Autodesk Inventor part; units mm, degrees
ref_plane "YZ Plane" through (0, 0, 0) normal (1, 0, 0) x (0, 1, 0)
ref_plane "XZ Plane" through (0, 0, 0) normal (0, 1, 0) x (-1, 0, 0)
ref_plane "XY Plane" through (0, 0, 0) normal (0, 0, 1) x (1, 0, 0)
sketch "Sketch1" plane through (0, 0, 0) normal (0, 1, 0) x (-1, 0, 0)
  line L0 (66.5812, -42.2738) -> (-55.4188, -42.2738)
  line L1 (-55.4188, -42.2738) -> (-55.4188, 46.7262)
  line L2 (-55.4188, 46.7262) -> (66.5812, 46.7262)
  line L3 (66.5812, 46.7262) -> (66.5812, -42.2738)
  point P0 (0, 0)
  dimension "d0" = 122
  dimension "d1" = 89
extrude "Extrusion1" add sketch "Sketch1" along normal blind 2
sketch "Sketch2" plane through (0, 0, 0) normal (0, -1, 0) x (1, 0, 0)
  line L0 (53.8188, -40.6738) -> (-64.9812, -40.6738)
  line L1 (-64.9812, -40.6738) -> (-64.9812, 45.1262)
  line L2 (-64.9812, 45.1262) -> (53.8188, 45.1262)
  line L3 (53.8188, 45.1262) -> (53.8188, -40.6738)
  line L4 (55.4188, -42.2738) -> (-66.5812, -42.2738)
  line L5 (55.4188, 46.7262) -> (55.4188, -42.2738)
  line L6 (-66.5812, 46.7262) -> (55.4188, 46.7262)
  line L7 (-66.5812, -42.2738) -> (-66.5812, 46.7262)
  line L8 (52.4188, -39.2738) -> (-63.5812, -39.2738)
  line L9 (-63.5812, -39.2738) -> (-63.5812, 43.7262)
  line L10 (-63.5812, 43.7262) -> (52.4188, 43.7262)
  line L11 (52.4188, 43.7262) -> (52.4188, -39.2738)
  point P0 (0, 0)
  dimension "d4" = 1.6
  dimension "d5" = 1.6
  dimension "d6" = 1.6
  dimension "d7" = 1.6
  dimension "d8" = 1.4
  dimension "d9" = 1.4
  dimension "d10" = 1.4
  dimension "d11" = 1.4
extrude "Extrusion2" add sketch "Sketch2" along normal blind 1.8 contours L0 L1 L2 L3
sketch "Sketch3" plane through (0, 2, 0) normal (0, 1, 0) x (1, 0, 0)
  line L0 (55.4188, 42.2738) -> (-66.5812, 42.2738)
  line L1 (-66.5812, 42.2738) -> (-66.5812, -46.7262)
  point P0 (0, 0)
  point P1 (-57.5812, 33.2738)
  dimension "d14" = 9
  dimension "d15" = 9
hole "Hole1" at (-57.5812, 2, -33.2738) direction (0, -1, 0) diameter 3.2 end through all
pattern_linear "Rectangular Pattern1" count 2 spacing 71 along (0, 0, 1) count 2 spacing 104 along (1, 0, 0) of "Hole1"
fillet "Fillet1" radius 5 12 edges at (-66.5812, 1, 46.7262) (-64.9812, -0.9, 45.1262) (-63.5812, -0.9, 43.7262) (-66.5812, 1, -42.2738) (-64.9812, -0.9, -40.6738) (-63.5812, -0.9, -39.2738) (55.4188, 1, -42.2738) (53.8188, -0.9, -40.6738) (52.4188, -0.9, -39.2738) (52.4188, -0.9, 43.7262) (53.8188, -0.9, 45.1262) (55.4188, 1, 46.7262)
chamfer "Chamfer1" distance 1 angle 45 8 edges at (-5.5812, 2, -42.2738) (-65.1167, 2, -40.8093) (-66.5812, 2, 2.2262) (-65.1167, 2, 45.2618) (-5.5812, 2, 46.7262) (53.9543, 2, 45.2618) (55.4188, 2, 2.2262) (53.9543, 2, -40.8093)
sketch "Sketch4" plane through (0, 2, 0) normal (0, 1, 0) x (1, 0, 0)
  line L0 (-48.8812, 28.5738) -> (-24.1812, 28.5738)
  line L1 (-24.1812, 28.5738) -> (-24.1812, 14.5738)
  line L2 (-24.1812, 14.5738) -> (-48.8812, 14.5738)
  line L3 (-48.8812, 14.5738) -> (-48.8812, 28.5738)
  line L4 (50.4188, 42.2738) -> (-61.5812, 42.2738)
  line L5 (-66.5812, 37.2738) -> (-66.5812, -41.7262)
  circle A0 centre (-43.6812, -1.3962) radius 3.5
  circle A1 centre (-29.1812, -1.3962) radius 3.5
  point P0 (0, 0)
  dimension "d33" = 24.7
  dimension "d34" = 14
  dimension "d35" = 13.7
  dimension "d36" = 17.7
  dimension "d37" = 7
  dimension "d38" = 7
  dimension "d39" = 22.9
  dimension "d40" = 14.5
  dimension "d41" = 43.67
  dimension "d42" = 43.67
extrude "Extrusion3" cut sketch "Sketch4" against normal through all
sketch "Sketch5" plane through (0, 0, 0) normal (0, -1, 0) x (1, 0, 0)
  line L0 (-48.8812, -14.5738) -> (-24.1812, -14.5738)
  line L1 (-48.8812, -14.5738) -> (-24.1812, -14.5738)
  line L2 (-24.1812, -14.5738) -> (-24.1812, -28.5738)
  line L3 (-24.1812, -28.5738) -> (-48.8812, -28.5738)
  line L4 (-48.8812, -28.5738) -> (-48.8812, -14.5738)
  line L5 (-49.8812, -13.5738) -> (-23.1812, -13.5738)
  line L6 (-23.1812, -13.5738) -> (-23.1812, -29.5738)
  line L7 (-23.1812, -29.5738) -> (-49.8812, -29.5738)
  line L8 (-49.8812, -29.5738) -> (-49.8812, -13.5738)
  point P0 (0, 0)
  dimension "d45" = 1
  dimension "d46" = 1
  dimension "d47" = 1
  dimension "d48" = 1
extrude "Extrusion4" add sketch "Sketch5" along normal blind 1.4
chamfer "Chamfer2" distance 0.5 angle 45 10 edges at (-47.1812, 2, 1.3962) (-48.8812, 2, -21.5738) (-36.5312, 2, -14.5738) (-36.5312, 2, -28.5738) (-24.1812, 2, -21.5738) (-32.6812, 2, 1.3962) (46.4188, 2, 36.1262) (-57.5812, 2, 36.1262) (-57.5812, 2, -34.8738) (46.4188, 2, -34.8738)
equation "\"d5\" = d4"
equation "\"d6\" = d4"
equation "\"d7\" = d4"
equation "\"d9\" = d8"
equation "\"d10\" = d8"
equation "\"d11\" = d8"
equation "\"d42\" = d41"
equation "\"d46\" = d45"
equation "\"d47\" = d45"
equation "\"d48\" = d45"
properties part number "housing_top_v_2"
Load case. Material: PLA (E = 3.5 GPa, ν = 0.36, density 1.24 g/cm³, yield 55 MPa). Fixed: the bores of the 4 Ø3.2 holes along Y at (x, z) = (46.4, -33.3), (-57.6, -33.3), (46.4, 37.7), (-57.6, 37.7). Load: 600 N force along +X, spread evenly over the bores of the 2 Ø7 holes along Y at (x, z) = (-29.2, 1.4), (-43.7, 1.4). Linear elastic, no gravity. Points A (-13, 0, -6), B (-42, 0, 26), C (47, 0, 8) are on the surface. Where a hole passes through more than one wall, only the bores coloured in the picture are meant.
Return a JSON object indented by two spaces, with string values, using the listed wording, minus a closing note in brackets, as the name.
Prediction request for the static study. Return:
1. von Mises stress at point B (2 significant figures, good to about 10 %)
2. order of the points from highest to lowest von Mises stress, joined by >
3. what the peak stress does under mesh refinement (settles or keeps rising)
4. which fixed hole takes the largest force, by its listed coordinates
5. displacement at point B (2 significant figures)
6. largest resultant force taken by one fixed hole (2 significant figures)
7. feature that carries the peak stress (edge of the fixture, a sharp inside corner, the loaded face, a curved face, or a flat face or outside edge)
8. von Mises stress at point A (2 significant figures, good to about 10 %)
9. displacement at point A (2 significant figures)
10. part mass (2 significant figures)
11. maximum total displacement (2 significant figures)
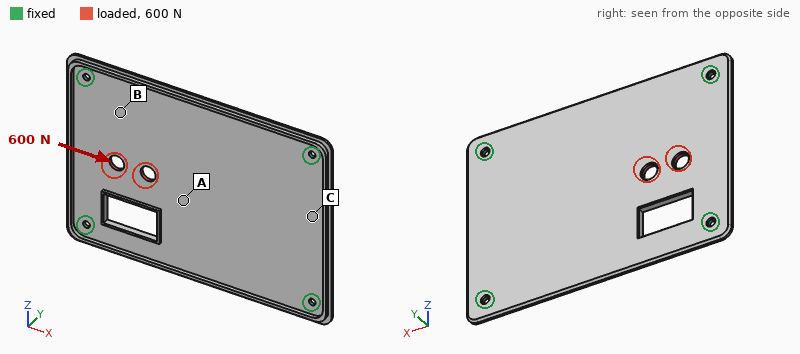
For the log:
{
  "von Mises stress at point B": "3.8 MPa",
  "order of the points from highest to lowest von Mises stress, joined by >": "A > B > C",
  "what the peak stress does under mesh refinement": "keeps rising",
  "which fixed hole takes the largest force, by its listed coordinates": "(-57.6, 37.7)",
  "displacement at point B": "0.054 mm",
  "largest resultant force taken by one fixed hole": "200 N",
  "feature that carries the peak stress": "edge of the fixture",
  "von Mises stress at point A": "5.8 MPa",
  "displacement at point A": "0.15 mm",
  "part mass": "27 g",
  "maximum total displacement": "0.18 mm"
}
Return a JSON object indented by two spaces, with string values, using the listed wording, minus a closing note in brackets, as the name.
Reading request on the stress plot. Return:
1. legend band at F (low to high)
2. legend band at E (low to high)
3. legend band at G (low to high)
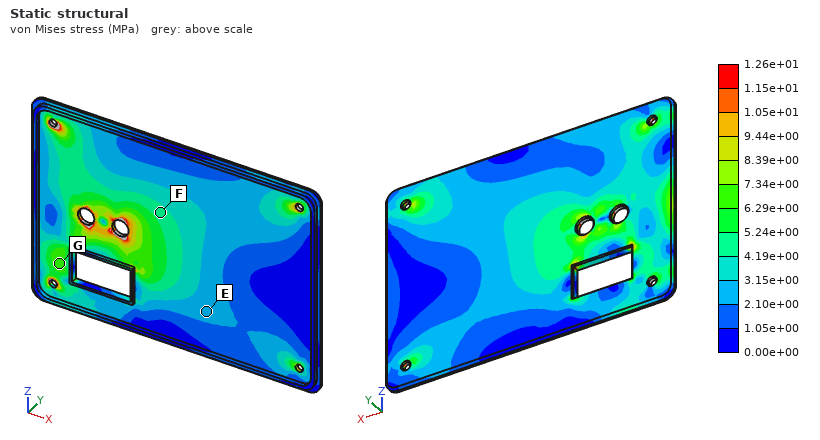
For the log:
{
  "legend band at F": "4.19e+00 to 5.24e+00 MPa",
  "legend band at E": "2.10e+00 to 3.15e+00 MPa",
  "legend band at G": "6.29e+00 to 7.34e+00 MPa"
}
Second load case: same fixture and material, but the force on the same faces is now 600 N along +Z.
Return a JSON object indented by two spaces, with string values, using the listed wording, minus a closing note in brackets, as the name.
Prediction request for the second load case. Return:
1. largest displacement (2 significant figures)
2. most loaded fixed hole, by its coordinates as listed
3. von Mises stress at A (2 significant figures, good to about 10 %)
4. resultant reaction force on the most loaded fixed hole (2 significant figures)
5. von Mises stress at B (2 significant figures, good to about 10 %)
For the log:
{
  "largest displacement": "0.17 mm",
  "most loaded fixed hole, by its coordinates as listed": "(-57.6, 37.7)",
  "von Mises stress at A": "2.4 MPa",
  "resultant reaction force on the most loaded fixed hole": "260 N",
  "von Mises stress at B": "5.6 MPa"
}
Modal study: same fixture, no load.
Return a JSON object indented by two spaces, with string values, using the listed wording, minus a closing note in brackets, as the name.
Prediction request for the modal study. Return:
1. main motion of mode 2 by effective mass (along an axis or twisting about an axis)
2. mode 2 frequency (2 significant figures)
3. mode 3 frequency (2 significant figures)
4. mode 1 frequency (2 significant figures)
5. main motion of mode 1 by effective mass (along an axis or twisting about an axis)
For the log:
{
  "main motion of mode 2 by effective mass": "twisting about X",
  "mode 2 frequency": "430 Hz",
  "mode 3 frequency": "630 Hz",
  "mode 1 frequency": "280 Hz",
  "main motion of mode 1 by effective mass": "along Y"
}
